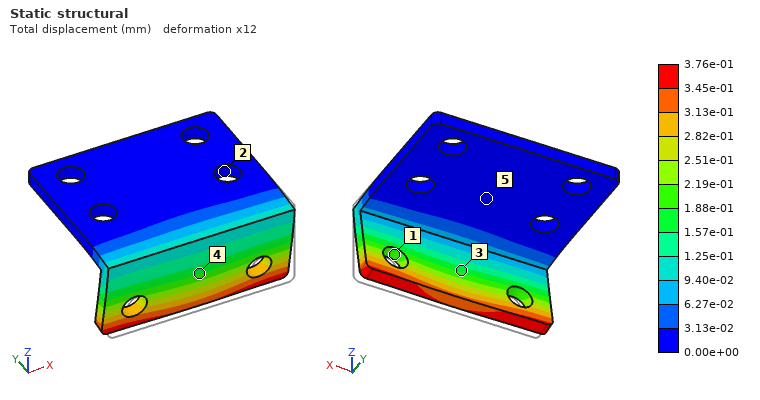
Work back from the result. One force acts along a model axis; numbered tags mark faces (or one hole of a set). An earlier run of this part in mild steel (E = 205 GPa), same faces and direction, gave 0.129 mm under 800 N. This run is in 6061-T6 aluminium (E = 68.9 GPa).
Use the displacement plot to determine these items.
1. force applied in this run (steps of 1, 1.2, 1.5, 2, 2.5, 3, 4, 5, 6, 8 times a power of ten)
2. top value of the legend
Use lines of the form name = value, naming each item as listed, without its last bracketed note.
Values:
force applied in this run = 800 N
top value of the legend = 3.76e-01 mm
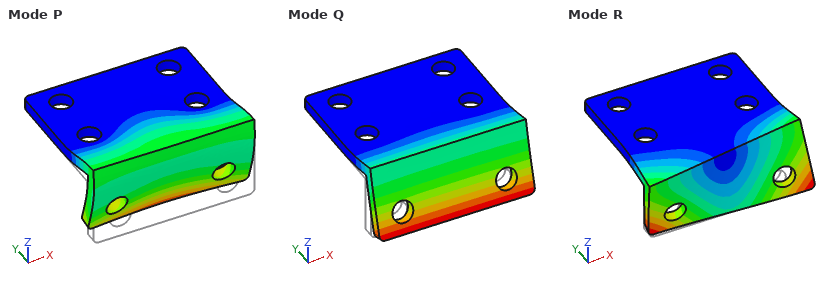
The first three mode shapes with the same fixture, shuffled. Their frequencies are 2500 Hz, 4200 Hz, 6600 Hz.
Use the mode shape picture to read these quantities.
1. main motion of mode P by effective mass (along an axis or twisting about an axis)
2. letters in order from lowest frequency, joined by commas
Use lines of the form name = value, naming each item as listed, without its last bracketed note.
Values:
main motion of mode P by effective mass = along Z
letters in order from lowest frequency, joined by commas = Q, R, P
